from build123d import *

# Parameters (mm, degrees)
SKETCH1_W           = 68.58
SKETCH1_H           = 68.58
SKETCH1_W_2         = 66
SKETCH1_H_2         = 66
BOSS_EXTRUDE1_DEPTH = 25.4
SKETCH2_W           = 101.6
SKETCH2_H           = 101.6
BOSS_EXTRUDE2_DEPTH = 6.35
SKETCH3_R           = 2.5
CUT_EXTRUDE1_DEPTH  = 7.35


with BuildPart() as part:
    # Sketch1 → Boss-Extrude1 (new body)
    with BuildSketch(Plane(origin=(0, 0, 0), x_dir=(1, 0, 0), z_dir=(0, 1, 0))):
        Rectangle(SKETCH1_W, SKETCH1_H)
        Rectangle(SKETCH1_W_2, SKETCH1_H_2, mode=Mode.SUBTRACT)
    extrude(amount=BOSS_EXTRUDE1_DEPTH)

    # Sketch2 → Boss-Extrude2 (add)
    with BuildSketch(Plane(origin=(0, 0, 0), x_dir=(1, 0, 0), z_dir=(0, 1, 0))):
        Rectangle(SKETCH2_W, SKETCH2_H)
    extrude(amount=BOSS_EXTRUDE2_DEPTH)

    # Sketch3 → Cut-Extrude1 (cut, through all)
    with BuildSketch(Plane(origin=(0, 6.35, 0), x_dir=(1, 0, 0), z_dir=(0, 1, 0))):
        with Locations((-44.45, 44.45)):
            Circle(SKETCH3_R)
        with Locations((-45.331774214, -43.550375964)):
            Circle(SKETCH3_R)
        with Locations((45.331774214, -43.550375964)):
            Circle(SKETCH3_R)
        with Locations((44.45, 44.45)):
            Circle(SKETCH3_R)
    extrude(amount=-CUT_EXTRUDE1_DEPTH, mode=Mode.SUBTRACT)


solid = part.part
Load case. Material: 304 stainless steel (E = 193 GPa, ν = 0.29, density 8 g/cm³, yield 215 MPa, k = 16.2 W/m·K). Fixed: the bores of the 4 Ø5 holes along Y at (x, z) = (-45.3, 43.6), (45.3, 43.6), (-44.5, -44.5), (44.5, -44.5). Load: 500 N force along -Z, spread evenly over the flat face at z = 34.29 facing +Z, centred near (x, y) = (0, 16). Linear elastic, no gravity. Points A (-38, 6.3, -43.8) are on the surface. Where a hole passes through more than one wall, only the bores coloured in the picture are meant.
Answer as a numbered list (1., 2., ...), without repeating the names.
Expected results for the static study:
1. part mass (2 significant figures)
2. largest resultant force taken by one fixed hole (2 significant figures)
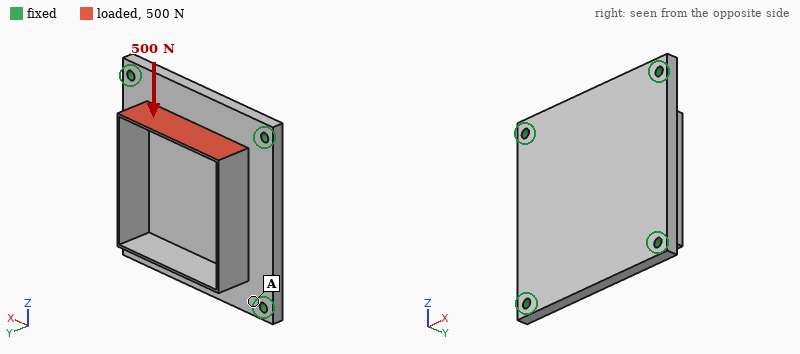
1. 570 g
2. 140 N
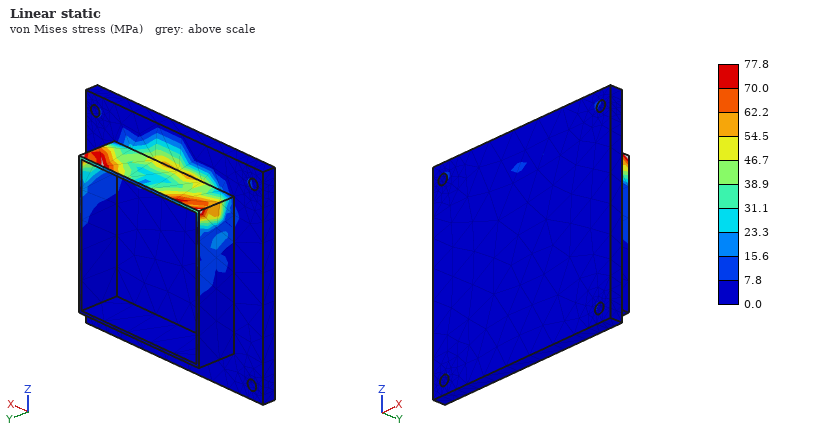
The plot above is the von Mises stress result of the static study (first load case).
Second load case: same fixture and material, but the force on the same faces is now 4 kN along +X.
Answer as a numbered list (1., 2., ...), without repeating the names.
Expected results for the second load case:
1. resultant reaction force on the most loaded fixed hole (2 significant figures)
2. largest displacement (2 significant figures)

1. 1.8 kN
2. 14 µm
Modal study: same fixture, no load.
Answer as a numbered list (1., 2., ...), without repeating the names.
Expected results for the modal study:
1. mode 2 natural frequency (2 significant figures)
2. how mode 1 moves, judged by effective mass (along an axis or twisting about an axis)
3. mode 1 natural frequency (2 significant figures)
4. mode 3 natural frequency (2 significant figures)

1. 3500 Hz
2. along Y
3. 3100 Hz
4. 3700 Hz
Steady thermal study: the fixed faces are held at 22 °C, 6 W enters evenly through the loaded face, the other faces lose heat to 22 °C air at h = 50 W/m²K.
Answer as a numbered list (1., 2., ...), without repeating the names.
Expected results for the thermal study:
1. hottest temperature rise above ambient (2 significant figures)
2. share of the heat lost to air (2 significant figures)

1. 32 K
2. 79 %
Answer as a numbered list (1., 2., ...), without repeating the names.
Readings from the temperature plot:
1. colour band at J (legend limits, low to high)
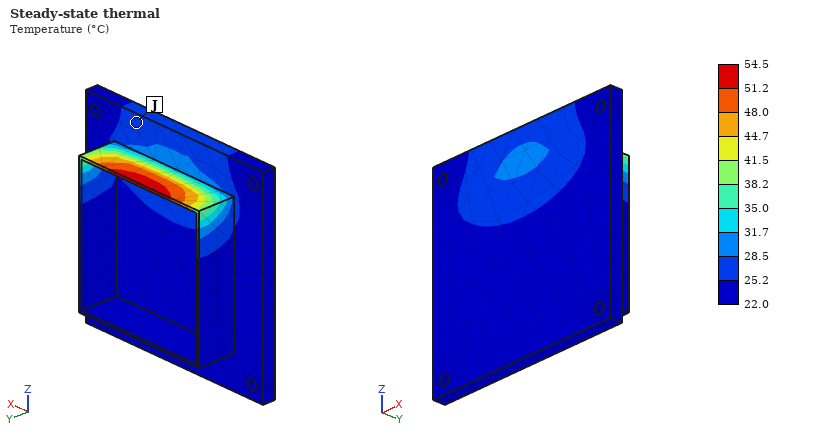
1. 25.2 to 28.5 °C
